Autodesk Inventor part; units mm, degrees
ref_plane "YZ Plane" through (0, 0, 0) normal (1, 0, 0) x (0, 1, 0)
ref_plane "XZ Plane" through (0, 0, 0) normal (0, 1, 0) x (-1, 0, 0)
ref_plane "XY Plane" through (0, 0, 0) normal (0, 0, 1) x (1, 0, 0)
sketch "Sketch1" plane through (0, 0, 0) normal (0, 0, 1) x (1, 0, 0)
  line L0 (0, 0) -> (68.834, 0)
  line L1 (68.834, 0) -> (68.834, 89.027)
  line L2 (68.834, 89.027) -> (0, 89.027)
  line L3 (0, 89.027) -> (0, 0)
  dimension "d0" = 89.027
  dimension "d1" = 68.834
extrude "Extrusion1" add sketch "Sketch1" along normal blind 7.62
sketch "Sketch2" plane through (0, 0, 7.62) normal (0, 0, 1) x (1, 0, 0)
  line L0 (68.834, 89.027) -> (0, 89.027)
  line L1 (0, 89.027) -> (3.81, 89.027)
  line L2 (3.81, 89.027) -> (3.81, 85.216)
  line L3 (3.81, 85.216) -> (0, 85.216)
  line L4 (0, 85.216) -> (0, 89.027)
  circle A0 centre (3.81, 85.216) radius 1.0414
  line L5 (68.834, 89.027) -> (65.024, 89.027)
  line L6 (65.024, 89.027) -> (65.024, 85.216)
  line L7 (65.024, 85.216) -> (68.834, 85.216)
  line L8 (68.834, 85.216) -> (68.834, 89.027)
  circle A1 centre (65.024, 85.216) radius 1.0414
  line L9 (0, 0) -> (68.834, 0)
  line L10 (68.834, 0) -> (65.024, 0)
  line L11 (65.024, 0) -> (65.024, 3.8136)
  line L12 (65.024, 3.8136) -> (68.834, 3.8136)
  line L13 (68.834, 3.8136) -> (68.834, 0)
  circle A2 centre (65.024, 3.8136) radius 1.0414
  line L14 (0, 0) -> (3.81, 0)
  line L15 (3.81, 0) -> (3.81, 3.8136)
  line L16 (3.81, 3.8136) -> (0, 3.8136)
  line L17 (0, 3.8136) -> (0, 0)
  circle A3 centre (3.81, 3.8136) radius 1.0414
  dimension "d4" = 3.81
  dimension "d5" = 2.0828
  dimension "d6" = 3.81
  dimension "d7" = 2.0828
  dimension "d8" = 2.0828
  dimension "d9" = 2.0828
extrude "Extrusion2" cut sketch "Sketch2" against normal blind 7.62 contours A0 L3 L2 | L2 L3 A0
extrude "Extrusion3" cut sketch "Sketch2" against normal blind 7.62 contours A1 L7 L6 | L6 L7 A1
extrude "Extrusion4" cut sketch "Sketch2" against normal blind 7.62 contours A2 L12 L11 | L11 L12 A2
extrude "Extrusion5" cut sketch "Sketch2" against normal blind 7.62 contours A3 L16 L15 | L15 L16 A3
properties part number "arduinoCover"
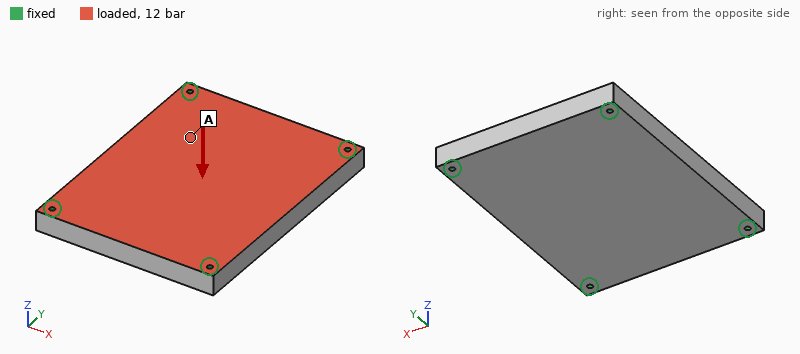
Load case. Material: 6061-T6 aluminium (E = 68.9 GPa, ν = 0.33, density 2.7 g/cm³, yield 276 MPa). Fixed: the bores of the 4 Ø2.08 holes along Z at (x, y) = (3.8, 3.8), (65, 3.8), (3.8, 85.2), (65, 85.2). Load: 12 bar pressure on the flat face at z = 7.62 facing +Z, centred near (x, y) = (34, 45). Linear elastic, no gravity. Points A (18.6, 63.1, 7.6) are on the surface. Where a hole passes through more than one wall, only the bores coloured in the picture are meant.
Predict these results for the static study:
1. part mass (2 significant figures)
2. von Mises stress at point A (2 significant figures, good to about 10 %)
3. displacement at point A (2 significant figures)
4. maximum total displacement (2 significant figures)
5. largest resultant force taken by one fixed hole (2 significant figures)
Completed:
130 g
32 MPa
0.10 mm
0.14 mm
1.8 kN
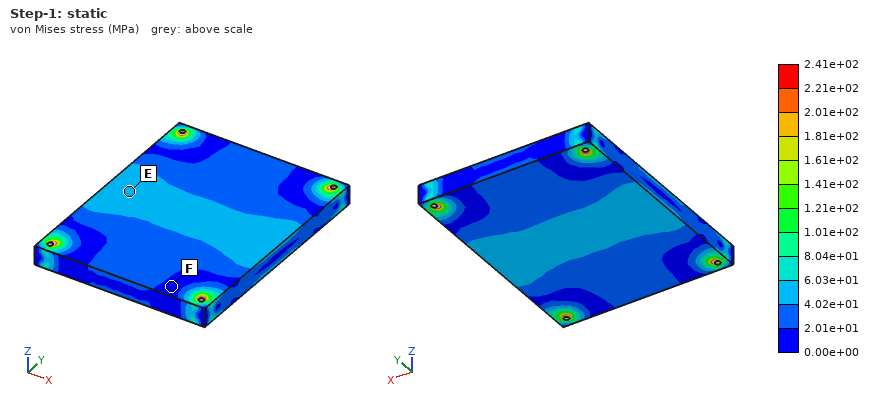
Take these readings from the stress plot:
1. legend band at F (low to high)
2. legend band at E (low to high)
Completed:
0.00e+00 to 2.01e+01 MPa
4.02e+01 to 6.03e+01 MPa
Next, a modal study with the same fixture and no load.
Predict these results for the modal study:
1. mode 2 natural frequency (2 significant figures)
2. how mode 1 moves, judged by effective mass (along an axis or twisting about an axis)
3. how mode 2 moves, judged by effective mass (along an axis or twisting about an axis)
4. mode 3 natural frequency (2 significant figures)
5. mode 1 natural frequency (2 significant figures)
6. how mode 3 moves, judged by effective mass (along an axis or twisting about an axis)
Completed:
6300 Hz
along Z
twisting about Y
8200 Hz
3800 Hz
twisting about X
